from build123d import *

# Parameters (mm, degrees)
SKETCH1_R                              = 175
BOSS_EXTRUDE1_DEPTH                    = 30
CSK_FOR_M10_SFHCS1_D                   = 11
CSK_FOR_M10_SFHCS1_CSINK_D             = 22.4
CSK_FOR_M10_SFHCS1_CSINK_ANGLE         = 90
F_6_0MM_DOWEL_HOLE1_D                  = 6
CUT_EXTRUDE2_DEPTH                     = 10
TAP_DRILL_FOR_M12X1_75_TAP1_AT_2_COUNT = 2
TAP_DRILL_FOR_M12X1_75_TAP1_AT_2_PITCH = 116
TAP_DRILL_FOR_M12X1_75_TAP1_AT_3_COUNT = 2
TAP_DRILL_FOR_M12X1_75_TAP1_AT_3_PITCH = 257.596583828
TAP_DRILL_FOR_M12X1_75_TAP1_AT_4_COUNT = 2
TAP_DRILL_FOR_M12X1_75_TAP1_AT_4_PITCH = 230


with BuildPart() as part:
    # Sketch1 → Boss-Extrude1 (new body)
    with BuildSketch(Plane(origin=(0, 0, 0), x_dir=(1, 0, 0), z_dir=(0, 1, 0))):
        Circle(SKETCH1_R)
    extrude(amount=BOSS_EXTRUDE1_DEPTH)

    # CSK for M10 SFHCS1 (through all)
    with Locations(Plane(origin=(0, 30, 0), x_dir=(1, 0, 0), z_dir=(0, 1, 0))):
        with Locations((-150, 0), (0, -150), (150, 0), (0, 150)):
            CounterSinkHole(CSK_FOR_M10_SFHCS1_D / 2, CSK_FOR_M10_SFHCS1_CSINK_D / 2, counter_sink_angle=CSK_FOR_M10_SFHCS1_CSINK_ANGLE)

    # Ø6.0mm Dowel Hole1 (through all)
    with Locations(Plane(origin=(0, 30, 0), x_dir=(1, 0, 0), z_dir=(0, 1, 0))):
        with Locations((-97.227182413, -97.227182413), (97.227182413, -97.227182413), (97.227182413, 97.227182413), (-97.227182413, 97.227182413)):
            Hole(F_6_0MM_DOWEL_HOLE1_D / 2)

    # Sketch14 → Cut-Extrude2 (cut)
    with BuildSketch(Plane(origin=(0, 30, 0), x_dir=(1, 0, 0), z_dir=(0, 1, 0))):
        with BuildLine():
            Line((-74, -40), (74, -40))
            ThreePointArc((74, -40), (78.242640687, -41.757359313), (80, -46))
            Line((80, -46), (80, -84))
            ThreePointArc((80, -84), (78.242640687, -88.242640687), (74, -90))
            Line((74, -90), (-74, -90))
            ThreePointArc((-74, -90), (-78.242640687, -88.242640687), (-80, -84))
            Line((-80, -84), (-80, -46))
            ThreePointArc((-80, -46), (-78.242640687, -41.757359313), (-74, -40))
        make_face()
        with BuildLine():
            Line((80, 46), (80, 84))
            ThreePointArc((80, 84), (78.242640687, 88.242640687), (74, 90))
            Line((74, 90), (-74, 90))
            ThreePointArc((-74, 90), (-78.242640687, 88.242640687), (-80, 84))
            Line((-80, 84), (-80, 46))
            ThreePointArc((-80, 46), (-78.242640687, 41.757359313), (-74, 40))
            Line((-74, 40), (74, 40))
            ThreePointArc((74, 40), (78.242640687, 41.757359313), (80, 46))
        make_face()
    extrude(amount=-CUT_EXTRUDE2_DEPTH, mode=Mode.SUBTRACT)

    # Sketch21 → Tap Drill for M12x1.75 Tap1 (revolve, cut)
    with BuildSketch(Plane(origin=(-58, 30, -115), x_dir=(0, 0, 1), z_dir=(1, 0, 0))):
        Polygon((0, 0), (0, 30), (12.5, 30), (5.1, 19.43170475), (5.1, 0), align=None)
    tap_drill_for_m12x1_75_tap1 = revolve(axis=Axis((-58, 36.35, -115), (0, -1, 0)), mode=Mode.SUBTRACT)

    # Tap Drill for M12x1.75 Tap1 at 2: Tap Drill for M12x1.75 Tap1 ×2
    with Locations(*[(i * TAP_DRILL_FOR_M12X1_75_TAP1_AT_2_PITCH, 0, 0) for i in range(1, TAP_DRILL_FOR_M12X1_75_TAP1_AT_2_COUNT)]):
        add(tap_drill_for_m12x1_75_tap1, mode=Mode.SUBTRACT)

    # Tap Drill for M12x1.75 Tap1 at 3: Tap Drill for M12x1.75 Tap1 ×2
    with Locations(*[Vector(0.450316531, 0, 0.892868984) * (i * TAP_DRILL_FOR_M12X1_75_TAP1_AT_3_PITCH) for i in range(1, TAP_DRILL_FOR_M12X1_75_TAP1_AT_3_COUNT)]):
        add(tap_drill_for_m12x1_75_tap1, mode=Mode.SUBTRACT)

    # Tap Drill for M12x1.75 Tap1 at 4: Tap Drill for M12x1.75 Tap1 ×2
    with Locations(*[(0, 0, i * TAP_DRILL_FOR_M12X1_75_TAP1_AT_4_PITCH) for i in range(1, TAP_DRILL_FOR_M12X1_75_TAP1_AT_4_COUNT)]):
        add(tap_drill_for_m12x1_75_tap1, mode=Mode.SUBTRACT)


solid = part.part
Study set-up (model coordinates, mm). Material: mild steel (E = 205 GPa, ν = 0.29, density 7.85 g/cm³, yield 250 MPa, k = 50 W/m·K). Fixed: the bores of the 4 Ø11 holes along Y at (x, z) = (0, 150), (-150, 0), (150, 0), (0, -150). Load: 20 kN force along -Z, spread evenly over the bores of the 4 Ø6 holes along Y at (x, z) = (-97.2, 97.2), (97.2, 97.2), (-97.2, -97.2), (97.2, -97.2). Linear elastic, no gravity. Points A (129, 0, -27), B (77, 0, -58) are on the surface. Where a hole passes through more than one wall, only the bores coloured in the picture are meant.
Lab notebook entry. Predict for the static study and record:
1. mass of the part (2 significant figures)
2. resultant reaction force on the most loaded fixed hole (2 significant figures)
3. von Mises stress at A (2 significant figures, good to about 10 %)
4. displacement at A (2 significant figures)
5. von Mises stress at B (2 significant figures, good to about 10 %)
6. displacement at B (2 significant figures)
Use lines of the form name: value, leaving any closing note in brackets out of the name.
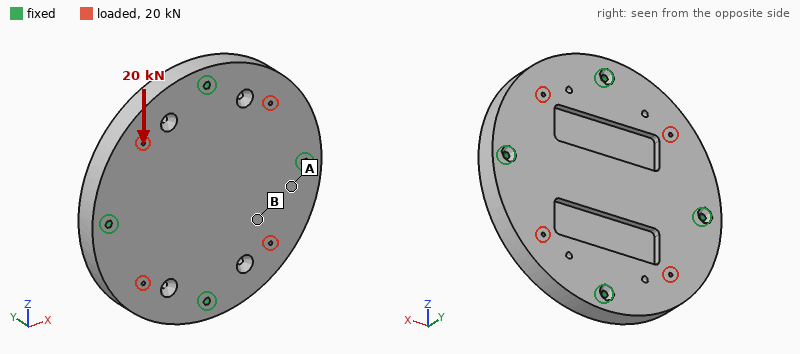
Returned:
mass of the part: 21 kg
resultant reaction force on the most loaded fixed hole: 5.8 kN
von Mises stress at A: 2.3 MPa
displacement at A: 0.63 µm
von Mises stress at B: 1.1 MPa
displacement at B: 1.1 µm
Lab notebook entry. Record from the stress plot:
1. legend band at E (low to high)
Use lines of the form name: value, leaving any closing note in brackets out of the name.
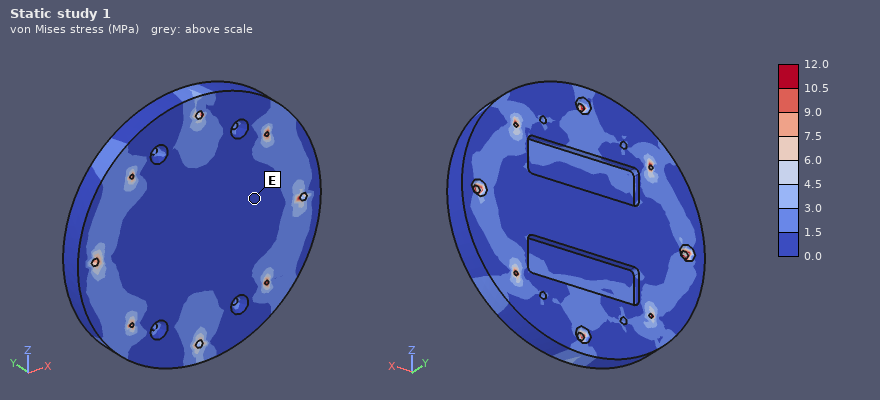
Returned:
legend band at E: 0.0 to 1.5 MPa
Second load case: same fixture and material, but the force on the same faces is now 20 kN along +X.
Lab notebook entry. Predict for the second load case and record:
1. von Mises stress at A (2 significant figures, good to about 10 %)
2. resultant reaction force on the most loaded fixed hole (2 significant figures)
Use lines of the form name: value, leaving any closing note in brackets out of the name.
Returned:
von Mises stress at A: 1.6 MPa
resultant reaction force on the most loaded fixed hole: 5.7 kN
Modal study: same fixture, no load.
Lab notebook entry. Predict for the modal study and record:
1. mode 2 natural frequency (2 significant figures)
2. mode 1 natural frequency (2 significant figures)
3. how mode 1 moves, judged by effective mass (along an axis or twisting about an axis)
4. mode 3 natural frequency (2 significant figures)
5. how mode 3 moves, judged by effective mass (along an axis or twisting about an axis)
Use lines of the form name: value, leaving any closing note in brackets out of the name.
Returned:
mode 2 natural frequency: 2000 Hz
mode 1 natural frequency: 1800 Hz
how mode 1 moves, judged by effective mass: along Y
mode 3 natural frequency: 2200 Hz
how mode 3 moves, judged by effective mass: twisting about X
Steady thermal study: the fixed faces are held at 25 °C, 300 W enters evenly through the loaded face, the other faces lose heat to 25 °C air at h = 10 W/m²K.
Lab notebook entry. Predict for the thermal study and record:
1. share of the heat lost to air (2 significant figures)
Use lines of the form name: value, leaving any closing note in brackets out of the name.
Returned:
share of the heat lost to air: 18 %
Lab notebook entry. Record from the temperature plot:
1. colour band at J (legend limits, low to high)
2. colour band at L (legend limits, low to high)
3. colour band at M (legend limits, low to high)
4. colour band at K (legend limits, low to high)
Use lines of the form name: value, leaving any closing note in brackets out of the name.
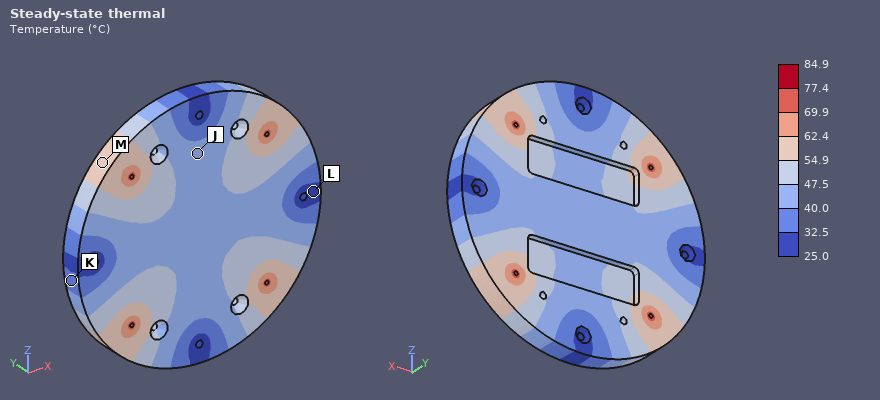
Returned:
colour band at J: 40.0 to 47.5 °C
colour band at L: 25.0 to 32.5 °C
colour band at M: 54.9 to 62.4 °C
colour band at K: 32.5 to 40.0 °C
